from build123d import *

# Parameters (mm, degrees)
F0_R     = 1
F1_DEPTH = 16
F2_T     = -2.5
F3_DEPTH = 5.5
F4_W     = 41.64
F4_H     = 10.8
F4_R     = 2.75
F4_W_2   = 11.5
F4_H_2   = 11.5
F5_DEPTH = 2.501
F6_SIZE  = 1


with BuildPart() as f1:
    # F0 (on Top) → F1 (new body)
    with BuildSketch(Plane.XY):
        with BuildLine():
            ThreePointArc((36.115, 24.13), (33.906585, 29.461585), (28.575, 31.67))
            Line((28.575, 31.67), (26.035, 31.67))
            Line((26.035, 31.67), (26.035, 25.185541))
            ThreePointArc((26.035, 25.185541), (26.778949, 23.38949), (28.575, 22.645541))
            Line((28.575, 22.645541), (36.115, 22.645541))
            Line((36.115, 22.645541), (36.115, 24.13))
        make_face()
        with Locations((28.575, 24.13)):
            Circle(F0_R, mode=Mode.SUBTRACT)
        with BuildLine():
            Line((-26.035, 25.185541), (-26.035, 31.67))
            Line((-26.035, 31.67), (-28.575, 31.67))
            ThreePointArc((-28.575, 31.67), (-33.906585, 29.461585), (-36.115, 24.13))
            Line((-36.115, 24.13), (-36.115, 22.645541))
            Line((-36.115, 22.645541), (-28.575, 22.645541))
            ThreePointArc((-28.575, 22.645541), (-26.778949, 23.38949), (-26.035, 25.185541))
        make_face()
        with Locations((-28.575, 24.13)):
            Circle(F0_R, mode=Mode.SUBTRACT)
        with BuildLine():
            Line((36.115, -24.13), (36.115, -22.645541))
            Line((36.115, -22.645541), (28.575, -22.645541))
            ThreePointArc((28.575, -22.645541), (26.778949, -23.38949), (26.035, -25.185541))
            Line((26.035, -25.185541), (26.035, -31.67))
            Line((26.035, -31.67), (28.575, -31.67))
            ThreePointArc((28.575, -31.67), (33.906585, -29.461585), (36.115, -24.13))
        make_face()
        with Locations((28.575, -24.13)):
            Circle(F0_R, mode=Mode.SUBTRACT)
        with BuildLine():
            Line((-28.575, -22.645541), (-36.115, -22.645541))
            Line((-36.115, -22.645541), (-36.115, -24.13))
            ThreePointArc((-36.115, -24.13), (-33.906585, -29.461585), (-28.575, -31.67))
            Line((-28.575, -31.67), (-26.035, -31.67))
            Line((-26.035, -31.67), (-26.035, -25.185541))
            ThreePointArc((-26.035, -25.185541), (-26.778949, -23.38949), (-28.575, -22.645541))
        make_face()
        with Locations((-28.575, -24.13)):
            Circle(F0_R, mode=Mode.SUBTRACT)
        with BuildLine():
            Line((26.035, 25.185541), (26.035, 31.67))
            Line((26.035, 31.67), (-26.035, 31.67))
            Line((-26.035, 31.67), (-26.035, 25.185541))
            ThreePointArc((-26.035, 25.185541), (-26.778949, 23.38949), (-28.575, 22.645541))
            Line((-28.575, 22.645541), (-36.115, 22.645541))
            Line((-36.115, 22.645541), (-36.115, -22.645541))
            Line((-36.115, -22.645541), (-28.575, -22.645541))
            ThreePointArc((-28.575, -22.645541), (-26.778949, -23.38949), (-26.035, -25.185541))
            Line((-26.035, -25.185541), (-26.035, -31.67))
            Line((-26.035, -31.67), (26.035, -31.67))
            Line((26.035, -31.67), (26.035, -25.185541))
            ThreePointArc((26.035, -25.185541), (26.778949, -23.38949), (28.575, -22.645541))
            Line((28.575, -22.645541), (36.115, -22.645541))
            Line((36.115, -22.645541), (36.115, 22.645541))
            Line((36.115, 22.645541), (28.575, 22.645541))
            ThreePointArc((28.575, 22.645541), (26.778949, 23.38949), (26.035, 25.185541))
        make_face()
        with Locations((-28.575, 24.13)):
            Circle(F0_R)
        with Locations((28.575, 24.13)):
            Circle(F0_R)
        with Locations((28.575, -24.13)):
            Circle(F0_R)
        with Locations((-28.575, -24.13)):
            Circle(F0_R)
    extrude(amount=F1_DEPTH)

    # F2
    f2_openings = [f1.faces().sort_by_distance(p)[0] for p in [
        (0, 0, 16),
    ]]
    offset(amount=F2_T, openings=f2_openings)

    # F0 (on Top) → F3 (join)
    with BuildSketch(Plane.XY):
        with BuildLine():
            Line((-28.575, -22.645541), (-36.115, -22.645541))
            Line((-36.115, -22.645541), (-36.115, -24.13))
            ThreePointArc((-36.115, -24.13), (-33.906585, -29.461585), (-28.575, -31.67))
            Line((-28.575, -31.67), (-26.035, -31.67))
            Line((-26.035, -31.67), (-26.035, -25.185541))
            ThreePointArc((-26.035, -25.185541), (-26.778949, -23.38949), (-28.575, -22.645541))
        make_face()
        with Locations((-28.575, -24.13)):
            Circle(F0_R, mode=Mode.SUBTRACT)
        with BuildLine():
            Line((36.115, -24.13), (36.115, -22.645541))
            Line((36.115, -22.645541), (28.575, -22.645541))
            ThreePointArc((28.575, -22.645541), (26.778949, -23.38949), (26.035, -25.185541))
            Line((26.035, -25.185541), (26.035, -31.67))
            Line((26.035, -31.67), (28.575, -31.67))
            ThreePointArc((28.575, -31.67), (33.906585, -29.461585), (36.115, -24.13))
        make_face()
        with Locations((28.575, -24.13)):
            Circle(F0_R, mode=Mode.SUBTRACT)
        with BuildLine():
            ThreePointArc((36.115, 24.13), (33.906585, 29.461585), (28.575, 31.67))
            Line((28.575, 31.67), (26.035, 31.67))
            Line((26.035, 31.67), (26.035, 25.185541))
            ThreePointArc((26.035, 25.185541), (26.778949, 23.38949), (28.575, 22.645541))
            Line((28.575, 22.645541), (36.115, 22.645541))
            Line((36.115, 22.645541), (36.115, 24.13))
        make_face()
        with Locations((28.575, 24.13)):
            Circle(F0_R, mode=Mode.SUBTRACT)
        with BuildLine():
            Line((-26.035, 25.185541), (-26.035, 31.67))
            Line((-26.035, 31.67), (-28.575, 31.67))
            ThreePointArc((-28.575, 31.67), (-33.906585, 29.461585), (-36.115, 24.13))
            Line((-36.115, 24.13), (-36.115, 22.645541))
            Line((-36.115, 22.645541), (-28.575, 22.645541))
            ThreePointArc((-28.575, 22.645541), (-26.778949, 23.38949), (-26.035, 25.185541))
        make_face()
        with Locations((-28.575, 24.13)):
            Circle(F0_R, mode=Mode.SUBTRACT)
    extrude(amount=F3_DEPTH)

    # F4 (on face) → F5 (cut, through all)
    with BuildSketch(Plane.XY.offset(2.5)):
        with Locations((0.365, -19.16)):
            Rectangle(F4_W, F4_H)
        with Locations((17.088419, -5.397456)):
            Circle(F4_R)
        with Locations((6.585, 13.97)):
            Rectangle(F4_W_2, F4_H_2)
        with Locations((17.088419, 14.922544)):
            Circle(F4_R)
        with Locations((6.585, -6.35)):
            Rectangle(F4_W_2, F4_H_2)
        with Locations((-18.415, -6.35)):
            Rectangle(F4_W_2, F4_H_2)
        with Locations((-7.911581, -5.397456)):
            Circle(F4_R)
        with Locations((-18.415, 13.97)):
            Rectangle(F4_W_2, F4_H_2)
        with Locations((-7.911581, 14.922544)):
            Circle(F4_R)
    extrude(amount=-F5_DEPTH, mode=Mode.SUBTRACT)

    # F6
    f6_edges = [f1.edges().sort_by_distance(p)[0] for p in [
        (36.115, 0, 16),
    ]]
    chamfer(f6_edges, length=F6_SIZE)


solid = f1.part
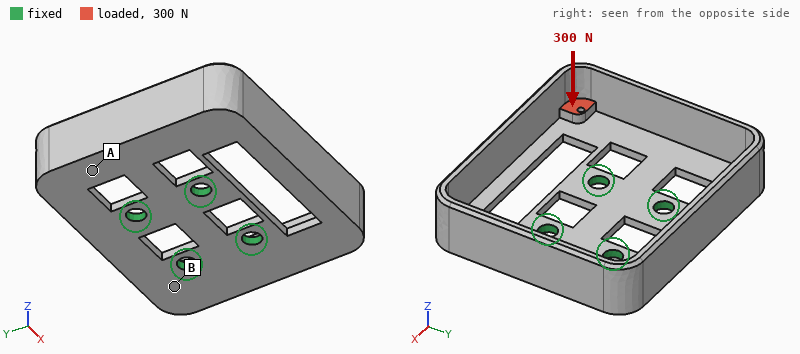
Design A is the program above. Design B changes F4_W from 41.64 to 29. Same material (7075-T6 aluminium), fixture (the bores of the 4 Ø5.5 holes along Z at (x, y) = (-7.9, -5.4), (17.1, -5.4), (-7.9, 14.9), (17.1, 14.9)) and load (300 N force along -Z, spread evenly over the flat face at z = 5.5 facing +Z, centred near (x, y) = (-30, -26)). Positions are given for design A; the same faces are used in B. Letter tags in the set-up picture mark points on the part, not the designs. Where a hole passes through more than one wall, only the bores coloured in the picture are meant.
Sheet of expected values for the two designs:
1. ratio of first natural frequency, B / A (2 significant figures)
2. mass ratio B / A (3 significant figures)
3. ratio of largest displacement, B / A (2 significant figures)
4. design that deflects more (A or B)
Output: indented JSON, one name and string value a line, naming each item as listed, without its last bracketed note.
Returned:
{
  "ratio of first natural frequency, B / A": "1.1",
  "mass ratio B / A": "1.02",
  "ratio of largest displacement, B / A": "0.81",
  "design that deflects more": "A"
}
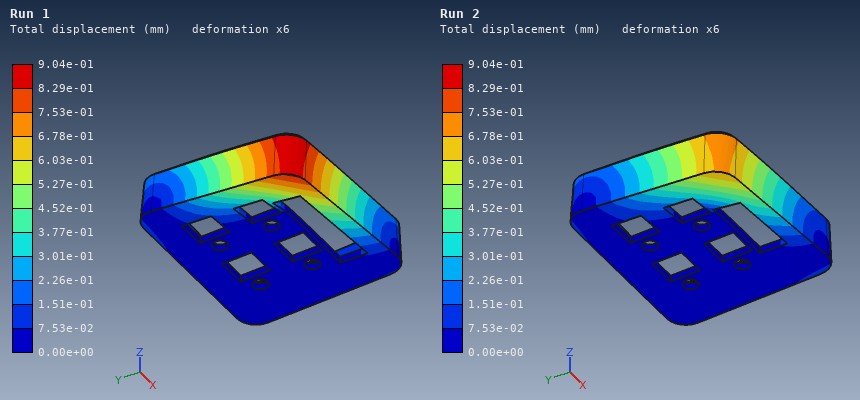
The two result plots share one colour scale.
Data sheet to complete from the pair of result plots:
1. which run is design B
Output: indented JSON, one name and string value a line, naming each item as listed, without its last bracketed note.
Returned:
{
  "which run is design B": "Run 2"
}
